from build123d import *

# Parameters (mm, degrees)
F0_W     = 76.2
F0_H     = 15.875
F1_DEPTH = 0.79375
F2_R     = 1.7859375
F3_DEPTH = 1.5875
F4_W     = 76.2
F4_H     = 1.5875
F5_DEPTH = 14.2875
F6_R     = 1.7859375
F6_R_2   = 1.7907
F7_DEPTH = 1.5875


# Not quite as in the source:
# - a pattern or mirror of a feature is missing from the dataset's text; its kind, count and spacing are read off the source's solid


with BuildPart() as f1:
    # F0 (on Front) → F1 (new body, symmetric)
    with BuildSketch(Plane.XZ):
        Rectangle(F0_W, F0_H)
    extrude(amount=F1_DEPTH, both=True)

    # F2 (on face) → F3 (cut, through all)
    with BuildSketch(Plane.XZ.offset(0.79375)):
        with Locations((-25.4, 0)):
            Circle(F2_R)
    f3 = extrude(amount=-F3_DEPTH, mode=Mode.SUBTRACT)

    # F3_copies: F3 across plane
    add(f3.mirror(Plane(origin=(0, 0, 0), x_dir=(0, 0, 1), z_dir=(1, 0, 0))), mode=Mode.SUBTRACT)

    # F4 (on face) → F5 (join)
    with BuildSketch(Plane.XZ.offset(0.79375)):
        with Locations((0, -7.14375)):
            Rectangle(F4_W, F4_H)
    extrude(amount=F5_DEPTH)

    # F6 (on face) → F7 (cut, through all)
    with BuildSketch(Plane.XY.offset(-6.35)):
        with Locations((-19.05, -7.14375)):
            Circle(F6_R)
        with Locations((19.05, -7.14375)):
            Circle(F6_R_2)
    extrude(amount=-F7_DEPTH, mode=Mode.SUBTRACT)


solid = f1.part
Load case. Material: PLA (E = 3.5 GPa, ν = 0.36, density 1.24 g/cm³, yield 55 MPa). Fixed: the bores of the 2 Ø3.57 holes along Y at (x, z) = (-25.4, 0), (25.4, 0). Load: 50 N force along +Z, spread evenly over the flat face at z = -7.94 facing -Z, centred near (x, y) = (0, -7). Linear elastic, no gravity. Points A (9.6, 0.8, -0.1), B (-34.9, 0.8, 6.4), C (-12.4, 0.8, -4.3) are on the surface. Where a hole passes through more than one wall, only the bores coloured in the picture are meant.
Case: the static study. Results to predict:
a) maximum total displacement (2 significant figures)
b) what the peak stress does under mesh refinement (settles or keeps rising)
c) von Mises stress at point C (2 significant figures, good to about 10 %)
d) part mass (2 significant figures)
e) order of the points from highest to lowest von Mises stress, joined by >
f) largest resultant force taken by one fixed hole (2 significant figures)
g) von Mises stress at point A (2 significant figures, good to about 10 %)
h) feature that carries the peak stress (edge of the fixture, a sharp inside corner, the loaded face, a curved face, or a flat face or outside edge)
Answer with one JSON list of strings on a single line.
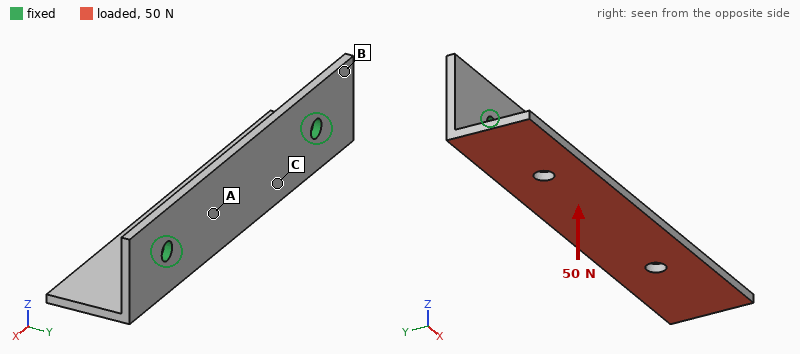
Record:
["0.87 mm", "keeps rising", "8.0 MPa", "4.4 g", "C > A > B", "25 N", "5.1 MPa", "edge of the fixture"]
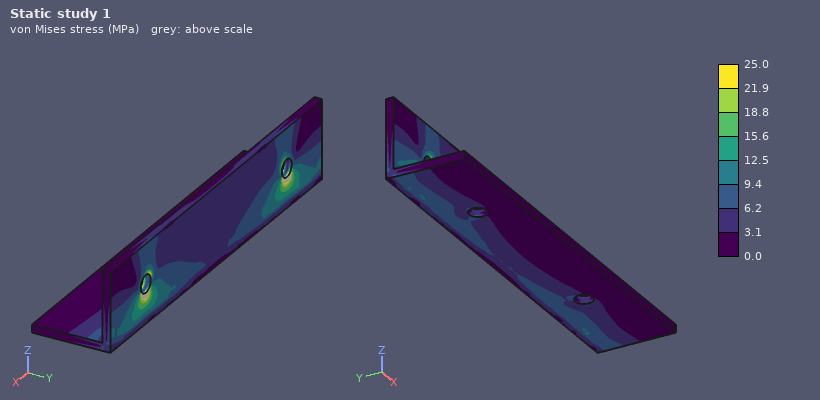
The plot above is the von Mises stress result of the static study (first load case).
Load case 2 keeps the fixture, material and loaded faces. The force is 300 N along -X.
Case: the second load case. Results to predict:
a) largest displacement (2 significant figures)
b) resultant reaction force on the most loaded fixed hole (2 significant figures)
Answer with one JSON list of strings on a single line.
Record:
["0.37 mm", "160 N"]
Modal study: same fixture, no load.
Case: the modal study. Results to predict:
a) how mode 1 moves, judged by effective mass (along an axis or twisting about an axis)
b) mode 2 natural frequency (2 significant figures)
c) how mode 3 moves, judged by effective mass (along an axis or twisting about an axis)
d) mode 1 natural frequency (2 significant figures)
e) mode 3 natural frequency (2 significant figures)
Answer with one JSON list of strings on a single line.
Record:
["along Z", "1300 Hz", "along Y", "940 Hz", "1600 Hz"]
